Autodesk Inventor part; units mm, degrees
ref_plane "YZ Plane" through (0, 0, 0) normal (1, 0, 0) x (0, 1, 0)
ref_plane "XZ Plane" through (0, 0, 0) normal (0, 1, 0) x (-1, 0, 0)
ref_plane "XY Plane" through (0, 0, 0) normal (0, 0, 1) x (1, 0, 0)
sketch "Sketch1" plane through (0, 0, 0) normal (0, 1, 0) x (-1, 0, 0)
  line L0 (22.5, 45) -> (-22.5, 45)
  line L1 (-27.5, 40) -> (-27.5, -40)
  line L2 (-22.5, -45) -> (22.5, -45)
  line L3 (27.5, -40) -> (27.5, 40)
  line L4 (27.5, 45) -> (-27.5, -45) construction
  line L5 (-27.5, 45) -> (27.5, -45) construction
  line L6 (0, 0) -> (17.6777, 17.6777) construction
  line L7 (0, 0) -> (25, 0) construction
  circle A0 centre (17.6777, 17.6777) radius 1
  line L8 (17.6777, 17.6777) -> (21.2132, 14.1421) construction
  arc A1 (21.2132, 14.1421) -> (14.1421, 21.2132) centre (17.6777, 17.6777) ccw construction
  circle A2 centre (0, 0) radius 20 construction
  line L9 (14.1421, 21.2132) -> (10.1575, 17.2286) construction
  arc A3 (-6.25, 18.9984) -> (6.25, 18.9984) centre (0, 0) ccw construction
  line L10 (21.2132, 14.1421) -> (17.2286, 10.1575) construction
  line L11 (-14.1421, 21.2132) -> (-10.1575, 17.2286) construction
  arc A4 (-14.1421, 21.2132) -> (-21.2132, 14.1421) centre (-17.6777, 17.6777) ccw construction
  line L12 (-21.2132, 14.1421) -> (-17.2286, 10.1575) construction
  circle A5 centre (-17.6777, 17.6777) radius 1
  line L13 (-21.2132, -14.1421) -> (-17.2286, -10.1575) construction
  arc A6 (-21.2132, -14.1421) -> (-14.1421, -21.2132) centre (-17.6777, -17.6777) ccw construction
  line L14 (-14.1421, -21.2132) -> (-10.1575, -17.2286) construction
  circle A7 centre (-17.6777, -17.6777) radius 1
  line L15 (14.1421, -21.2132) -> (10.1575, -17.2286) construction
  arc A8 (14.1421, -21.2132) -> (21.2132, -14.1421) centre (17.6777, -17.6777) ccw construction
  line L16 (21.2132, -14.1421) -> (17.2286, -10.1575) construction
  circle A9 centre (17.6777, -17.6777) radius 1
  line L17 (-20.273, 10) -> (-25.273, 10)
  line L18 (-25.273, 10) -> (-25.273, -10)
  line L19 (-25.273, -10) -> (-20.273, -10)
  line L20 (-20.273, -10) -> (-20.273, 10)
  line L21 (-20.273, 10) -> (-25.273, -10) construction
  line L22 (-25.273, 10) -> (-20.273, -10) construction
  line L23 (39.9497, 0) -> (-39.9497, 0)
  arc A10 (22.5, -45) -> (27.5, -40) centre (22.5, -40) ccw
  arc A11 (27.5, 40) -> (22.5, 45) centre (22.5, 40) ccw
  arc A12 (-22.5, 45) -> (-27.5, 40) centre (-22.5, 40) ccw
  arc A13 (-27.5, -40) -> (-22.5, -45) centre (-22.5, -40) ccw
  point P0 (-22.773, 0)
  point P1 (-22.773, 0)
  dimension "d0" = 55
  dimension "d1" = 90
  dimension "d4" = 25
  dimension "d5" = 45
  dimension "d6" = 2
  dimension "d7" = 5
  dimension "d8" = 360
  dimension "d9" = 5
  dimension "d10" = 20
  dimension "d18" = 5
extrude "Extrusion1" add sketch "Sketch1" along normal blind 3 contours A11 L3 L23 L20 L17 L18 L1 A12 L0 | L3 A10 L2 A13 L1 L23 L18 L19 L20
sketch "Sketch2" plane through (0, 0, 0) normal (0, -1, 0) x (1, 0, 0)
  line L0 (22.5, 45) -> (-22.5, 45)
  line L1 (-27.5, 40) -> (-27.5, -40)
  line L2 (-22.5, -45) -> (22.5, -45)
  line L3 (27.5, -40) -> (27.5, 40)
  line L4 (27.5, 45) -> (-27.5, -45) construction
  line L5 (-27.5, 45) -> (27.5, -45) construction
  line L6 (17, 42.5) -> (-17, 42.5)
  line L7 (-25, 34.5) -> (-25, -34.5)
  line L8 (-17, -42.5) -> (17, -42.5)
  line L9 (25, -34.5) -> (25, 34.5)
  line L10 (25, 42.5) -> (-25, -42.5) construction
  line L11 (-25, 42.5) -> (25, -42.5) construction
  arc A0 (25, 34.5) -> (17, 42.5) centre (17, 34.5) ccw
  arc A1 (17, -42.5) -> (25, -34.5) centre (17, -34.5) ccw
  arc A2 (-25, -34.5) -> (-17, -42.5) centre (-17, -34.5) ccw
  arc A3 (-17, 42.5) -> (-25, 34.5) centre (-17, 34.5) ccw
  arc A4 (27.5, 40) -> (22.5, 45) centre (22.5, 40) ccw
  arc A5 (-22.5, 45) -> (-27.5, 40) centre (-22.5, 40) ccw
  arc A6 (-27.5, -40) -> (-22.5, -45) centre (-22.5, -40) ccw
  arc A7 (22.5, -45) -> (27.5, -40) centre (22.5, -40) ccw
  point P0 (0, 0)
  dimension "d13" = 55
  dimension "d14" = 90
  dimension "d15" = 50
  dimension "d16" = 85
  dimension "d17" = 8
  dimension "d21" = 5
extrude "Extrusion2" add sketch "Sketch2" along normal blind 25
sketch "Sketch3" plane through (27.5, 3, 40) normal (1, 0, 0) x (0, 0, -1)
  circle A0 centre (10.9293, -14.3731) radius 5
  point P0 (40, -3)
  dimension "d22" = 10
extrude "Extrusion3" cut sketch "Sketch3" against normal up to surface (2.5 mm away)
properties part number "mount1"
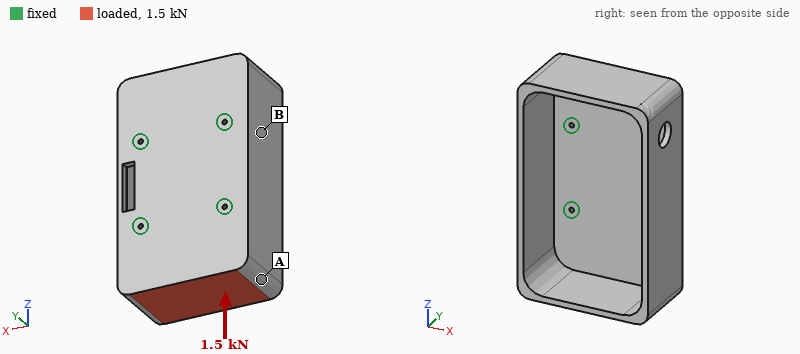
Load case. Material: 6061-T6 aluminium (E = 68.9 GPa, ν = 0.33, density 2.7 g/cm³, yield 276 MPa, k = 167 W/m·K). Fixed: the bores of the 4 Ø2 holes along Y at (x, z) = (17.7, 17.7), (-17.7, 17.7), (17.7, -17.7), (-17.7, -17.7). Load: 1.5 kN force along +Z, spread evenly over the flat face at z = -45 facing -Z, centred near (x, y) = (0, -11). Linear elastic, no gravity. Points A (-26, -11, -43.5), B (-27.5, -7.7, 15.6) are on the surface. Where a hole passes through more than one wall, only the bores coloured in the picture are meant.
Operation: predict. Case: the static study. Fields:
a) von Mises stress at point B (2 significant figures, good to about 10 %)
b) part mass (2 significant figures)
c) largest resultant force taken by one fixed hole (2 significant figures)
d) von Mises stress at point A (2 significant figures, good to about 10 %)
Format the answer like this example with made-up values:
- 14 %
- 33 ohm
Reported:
- 10 MPa
- 88 g
- 530 N
- 48 MPa
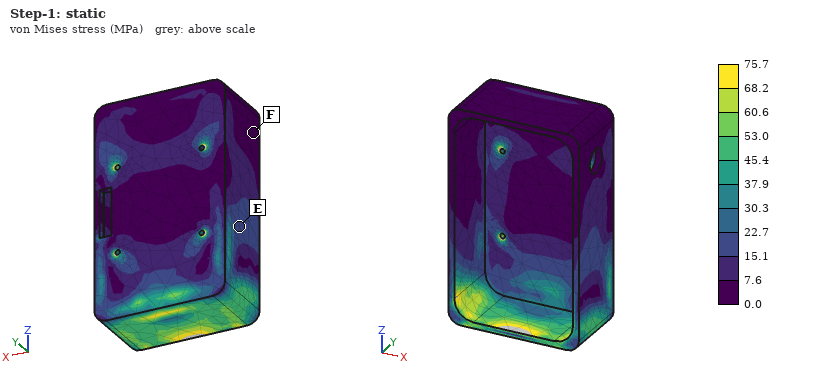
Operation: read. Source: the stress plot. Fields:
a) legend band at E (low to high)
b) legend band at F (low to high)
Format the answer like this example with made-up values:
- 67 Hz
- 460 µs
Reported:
- 15.1 to 22.7 MPa
- 0.0 to 7.6 MPa
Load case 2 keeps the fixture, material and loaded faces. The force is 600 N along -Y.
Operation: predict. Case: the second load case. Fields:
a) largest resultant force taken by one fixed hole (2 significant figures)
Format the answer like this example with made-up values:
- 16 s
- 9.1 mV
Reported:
- 510 N
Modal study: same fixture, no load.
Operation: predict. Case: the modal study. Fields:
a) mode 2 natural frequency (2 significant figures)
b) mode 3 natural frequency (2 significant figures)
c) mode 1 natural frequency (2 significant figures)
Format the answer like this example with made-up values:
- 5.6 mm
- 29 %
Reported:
- 2800 Hz
- 2800 Hz
- 2600 Hz
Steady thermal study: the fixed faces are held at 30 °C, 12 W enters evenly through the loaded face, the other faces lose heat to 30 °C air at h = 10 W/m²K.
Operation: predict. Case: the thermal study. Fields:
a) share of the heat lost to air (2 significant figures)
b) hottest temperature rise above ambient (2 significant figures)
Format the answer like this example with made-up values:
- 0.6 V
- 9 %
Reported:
- 6.2 %
- 13 K
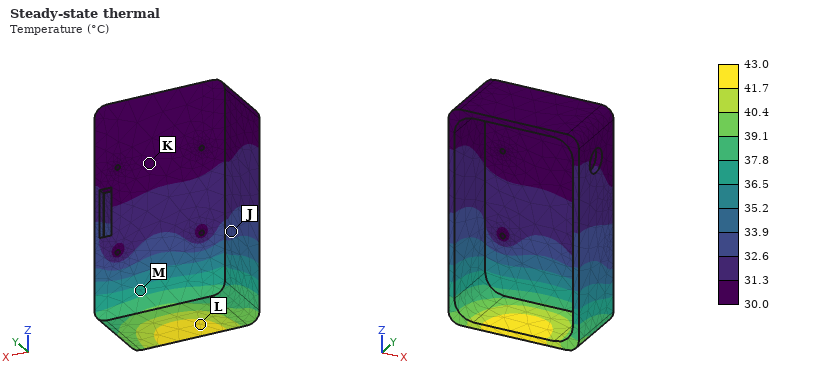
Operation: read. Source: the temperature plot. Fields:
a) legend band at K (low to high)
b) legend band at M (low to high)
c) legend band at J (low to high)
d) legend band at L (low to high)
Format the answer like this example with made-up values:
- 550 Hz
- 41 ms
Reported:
- 30.0 to 31.3 °C
- 36.5 to 37.8 °C
- 32.6 to 33.9 °C
- 41.7 to 43.0 °C
